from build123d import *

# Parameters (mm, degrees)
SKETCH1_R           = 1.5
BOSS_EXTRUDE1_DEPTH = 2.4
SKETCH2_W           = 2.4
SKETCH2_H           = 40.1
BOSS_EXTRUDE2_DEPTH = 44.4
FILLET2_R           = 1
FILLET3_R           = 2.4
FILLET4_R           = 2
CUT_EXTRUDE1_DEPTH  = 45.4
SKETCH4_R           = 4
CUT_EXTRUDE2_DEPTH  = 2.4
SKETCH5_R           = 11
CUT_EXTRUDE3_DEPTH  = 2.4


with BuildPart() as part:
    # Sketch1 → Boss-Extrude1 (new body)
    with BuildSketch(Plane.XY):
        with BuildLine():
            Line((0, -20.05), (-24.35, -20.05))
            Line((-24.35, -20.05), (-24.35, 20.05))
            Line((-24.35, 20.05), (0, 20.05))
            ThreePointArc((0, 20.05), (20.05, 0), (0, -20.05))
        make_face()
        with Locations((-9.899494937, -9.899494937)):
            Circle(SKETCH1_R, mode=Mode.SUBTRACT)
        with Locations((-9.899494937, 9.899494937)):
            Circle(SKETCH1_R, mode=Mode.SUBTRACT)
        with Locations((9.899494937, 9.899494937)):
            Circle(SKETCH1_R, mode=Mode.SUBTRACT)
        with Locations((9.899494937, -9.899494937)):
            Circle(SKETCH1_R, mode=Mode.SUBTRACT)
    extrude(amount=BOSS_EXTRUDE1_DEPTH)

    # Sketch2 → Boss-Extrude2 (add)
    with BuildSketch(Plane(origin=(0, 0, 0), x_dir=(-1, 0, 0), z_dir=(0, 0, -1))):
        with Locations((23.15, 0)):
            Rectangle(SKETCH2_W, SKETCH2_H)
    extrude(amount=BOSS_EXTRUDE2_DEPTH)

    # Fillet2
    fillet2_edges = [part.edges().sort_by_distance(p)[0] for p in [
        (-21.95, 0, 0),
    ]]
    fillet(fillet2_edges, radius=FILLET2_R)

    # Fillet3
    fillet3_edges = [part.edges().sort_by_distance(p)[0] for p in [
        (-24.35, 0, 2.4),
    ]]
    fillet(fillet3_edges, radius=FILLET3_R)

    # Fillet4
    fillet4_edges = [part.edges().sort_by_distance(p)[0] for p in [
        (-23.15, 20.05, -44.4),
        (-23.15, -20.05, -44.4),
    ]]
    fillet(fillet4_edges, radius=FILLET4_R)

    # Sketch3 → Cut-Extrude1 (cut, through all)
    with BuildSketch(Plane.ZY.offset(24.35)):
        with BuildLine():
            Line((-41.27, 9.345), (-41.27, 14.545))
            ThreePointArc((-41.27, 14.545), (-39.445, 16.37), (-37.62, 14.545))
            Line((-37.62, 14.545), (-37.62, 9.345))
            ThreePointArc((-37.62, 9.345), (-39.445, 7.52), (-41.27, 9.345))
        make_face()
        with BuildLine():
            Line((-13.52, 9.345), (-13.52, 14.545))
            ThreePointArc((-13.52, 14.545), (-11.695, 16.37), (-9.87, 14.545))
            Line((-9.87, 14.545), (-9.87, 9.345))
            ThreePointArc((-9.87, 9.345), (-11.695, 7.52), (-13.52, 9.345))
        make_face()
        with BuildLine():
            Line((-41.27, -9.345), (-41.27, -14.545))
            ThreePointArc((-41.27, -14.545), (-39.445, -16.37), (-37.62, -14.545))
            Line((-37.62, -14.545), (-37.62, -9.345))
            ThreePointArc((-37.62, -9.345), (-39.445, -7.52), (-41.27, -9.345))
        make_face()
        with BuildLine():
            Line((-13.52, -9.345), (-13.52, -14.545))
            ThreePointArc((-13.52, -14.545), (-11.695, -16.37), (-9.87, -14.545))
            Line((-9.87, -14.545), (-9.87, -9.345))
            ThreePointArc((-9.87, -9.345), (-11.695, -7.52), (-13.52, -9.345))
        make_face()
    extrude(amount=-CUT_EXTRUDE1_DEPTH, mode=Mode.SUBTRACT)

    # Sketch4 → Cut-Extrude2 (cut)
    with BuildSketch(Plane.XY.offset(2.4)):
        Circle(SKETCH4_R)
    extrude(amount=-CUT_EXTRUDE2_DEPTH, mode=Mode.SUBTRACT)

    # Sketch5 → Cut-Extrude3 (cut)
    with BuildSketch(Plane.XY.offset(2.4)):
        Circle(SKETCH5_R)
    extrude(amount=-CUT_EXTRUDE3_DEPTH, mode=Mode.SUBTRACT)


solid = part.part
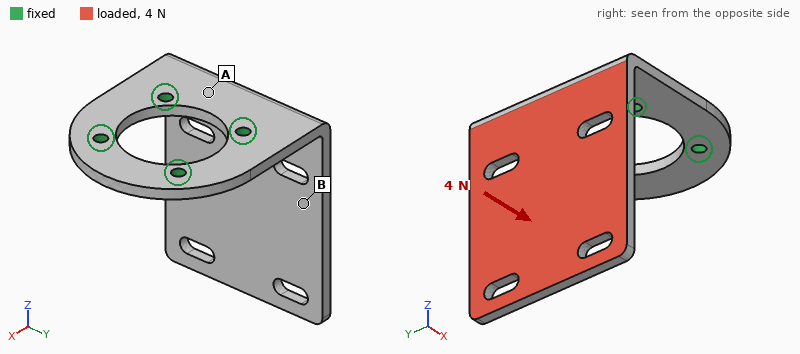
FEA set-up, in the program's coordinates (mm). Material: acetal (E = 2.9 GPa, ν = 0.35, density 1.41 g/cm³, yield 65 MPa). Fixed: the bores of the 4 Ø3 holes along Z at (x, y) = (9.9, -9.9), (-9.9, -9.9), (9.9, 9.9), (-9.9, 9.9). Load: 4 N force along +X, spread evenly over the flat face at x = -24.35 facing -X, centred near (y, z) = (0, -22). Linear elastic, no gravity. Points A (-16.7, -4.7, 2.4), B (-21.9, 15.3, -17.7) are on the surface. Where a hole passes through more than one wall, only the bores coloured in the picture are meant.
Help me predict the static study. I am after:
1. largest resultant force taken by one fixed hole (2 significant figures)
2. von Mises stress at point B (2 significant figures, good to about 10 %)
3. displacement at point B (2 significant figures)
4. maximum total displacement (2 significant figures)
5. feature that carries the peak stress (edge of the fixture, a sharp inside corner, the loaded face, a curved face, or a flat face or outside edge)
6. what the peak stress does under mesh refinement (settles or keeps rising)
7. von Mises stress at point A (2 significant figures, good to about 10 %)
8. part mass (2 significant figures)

2.2 N
0.71 MPa
0.26 mm
0.79 mm
edge of the fixture
keeps rising
2.0 MPa
9.6 g
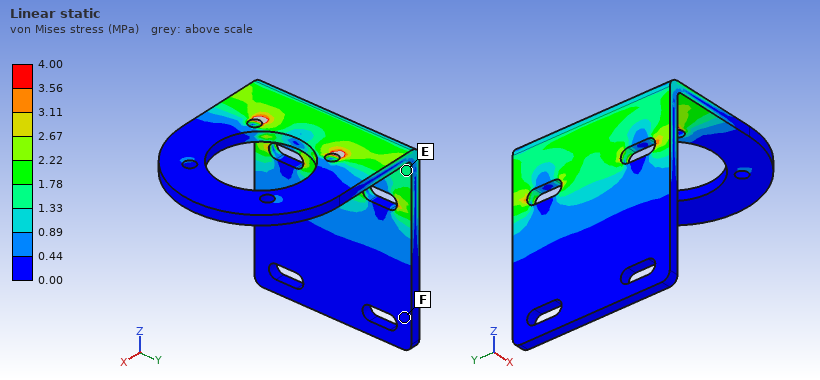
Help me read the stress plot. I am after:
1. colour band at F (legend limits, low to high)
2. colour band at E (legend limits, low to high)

0.00 to 0.44 MPa
1.33 to 1.78 MPa
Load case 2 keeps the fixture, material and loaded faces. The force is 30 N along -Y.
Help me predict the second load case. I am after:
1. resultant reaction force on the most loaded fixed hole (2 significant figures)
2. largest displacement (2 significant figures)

36 N
0.74 mm
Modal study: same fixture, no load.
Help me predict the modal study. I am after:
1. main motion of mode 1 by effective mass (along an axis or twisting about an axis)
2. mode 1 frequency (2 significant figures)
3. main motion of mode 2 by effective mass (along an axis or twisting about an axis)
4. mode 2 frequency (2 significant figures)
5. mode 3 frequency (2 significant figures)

along X
190 Hz
along Y
470 Hz
720 Hz
